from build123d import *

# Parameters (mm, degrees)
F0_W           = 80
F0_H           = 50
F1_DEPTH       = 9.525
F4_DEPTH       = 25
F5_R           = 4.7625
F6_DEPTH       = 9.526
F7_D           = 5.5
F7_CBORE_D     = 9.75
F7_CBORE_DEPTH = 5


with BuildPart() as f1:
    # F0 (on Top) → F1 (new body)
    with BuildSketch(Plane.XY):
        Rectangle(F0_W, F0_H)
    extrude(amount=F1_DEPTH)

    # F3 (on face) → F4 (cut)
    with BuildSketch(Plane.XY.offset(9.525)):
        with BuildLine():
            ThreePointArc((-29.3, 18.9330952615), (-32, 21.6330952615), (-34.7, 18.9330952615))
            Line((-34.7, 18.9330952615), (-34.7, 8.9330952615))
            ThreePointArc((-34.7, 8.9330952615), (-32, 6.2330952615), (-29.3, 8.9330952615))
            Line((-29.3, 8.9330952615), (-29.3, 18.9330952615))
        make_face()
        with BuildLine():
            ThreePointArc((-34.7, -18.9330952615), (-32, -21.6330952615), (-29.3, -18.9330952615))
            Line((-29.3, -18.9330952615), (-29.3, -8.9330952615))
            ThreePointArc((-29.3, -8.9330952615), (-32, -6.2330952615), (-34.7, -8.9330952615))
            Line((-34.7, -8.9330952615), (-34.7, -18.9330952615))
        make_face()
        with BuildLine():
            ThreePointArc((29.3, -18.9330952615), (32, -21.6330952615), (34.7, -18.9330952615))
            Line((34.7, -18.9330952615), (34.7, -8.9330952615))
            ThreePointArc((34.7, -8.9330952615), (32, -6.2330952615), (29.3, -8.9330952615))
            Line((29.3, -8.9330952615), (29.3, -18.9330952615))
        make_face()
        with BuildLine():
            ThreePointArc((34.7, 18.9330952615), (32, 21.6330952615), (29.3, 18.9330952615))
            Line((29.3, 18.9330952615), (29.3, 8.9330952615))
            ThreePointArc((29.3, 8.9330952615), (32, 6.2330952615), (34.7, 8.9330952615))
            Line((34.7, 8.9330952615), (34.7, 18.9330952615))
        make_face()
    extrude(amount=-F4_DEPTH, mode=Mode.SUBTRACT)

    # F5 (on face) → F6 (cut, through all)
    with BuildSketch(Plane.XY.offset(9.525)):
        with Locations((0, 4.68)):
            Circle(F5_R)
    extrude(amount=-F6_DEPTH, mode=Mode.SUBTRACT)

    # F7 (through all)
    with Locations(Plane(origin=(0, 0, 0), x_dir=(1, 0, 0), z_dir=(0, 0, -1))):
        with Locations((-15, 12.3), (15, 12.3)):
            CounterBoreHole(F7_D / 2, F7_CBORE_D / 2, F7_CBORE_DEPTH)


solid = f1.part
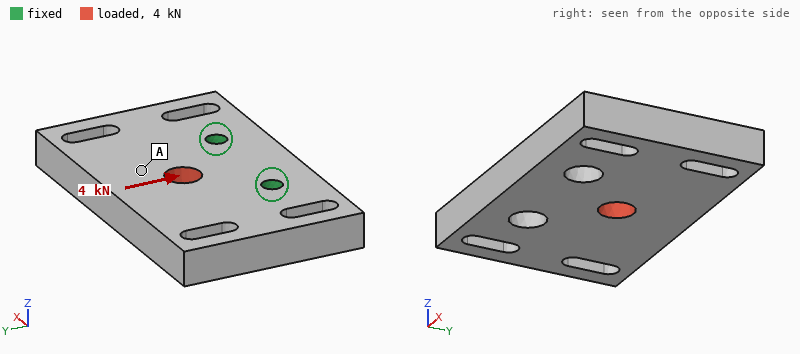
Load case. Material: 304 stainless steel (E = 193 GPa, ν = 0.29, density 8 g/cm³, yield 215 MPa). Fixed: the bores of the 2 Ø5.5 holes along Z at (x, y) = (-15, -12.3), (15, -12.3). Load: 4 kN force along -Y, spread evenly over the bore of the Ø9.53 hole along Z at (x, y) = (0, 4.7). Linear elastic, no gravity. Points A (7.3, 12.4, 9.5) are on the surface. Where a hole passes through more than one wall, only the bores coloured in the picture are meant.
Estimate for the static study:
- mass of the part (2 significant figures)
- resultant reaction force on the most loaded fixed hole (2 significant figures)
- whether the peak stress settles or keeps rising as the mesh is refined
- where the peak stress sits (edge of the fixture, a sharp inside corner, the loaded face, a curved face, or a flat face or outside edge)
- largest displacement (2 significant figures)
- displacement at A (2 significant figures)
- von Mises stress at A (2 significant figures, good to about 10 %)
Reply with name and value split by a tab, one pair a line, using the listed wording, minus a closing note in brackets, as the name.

mass of the part	270 g
resultant reaction force on the most loaded fixed hole	2.0 kN
whether the peak stress settles or keeps rising as the mesh is refined	keeps rising
where the peak stress sits	edge of the fixture
largest displacement	11 µm
displacement at A	7.0 µm
von Mises stress at A	9.5 MPa
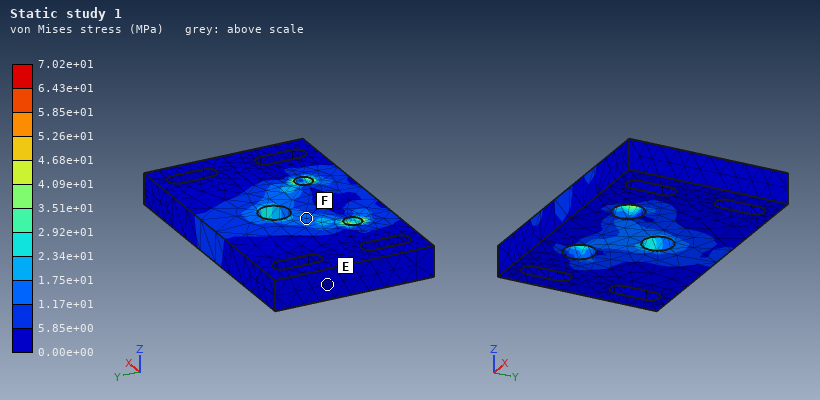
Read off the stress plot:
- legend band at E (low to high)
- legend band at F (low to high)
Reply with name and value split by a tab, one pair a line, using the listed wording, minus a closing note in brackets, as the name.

legend band at E	0.00e+00 to 5.85e+00 MPa
legend band at F	1.17e+01 to 1.75e+01 MPa
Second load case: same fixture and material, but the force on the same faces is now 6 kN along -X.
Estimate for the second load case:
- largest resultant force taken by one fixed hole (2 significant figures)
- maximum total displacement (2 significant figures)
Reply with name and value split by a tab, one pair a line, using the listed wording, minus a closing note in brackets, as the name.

largest resultant force taken by one fixed hole	4.3 kN
maximum total displacement	11 µm
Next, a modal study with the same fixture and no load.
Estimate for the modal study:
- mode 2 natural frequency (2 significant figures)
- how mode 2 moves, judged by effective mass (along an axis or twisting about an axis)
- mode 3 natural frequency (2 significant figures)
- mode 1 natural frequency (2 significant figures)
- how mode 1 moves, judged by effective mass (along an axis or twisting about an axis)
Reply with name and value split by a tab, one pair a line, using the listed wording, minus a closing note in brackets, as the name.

mode 2 natural frequency	4500 Hz
how mode 2 moves, judged by effective mass	twisting about Y
mode 3 natural frequency	7700 Hz
mode 1 natural frequency	2700 Hz
how mode 1 moves, judged by effective mass	along Z
